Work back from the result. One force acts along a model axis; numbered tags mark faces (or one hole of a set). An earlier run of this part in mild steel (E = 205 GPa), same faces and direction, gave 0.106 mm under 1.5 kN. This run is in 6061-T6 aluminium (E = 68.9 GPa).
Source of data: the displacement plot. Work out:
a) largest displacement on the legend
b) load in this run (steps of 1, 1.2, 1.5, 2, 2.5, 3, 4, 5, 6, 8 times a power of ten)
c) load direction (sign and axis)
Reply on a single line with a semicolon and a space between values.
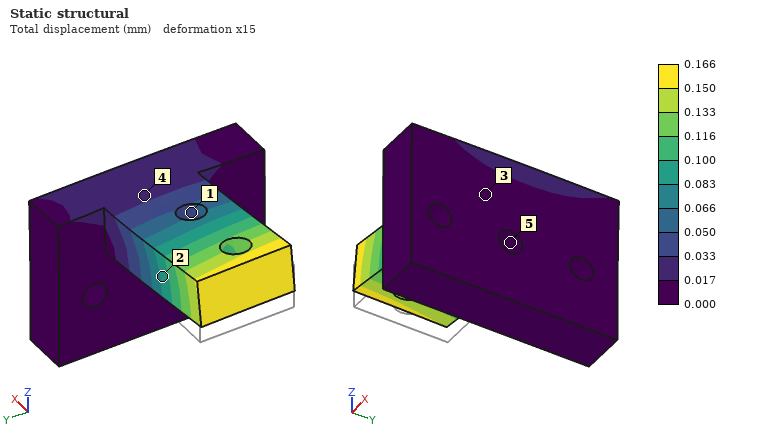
0.166 mm; 800 N; +Z
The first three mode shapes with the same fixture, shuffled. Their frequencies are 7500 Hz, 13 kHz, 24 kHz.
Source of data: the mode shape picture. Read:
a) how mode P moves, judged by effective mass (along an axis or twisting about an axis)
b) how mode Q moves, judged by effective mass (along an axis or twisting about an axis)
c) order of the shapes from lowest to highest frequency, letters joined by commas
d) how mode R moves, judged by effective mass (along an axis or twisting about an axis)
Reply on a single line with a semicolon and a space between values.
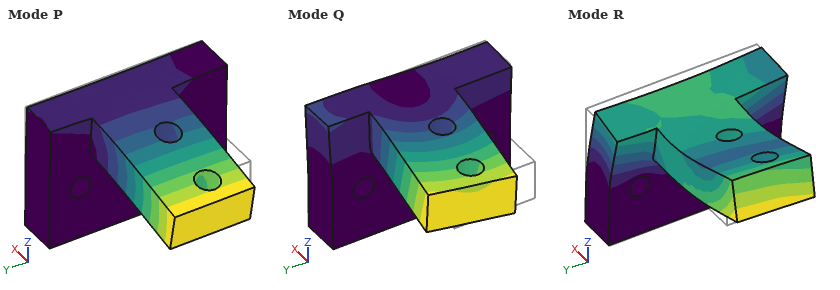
along Z; along Y; P, Q, R; along X
